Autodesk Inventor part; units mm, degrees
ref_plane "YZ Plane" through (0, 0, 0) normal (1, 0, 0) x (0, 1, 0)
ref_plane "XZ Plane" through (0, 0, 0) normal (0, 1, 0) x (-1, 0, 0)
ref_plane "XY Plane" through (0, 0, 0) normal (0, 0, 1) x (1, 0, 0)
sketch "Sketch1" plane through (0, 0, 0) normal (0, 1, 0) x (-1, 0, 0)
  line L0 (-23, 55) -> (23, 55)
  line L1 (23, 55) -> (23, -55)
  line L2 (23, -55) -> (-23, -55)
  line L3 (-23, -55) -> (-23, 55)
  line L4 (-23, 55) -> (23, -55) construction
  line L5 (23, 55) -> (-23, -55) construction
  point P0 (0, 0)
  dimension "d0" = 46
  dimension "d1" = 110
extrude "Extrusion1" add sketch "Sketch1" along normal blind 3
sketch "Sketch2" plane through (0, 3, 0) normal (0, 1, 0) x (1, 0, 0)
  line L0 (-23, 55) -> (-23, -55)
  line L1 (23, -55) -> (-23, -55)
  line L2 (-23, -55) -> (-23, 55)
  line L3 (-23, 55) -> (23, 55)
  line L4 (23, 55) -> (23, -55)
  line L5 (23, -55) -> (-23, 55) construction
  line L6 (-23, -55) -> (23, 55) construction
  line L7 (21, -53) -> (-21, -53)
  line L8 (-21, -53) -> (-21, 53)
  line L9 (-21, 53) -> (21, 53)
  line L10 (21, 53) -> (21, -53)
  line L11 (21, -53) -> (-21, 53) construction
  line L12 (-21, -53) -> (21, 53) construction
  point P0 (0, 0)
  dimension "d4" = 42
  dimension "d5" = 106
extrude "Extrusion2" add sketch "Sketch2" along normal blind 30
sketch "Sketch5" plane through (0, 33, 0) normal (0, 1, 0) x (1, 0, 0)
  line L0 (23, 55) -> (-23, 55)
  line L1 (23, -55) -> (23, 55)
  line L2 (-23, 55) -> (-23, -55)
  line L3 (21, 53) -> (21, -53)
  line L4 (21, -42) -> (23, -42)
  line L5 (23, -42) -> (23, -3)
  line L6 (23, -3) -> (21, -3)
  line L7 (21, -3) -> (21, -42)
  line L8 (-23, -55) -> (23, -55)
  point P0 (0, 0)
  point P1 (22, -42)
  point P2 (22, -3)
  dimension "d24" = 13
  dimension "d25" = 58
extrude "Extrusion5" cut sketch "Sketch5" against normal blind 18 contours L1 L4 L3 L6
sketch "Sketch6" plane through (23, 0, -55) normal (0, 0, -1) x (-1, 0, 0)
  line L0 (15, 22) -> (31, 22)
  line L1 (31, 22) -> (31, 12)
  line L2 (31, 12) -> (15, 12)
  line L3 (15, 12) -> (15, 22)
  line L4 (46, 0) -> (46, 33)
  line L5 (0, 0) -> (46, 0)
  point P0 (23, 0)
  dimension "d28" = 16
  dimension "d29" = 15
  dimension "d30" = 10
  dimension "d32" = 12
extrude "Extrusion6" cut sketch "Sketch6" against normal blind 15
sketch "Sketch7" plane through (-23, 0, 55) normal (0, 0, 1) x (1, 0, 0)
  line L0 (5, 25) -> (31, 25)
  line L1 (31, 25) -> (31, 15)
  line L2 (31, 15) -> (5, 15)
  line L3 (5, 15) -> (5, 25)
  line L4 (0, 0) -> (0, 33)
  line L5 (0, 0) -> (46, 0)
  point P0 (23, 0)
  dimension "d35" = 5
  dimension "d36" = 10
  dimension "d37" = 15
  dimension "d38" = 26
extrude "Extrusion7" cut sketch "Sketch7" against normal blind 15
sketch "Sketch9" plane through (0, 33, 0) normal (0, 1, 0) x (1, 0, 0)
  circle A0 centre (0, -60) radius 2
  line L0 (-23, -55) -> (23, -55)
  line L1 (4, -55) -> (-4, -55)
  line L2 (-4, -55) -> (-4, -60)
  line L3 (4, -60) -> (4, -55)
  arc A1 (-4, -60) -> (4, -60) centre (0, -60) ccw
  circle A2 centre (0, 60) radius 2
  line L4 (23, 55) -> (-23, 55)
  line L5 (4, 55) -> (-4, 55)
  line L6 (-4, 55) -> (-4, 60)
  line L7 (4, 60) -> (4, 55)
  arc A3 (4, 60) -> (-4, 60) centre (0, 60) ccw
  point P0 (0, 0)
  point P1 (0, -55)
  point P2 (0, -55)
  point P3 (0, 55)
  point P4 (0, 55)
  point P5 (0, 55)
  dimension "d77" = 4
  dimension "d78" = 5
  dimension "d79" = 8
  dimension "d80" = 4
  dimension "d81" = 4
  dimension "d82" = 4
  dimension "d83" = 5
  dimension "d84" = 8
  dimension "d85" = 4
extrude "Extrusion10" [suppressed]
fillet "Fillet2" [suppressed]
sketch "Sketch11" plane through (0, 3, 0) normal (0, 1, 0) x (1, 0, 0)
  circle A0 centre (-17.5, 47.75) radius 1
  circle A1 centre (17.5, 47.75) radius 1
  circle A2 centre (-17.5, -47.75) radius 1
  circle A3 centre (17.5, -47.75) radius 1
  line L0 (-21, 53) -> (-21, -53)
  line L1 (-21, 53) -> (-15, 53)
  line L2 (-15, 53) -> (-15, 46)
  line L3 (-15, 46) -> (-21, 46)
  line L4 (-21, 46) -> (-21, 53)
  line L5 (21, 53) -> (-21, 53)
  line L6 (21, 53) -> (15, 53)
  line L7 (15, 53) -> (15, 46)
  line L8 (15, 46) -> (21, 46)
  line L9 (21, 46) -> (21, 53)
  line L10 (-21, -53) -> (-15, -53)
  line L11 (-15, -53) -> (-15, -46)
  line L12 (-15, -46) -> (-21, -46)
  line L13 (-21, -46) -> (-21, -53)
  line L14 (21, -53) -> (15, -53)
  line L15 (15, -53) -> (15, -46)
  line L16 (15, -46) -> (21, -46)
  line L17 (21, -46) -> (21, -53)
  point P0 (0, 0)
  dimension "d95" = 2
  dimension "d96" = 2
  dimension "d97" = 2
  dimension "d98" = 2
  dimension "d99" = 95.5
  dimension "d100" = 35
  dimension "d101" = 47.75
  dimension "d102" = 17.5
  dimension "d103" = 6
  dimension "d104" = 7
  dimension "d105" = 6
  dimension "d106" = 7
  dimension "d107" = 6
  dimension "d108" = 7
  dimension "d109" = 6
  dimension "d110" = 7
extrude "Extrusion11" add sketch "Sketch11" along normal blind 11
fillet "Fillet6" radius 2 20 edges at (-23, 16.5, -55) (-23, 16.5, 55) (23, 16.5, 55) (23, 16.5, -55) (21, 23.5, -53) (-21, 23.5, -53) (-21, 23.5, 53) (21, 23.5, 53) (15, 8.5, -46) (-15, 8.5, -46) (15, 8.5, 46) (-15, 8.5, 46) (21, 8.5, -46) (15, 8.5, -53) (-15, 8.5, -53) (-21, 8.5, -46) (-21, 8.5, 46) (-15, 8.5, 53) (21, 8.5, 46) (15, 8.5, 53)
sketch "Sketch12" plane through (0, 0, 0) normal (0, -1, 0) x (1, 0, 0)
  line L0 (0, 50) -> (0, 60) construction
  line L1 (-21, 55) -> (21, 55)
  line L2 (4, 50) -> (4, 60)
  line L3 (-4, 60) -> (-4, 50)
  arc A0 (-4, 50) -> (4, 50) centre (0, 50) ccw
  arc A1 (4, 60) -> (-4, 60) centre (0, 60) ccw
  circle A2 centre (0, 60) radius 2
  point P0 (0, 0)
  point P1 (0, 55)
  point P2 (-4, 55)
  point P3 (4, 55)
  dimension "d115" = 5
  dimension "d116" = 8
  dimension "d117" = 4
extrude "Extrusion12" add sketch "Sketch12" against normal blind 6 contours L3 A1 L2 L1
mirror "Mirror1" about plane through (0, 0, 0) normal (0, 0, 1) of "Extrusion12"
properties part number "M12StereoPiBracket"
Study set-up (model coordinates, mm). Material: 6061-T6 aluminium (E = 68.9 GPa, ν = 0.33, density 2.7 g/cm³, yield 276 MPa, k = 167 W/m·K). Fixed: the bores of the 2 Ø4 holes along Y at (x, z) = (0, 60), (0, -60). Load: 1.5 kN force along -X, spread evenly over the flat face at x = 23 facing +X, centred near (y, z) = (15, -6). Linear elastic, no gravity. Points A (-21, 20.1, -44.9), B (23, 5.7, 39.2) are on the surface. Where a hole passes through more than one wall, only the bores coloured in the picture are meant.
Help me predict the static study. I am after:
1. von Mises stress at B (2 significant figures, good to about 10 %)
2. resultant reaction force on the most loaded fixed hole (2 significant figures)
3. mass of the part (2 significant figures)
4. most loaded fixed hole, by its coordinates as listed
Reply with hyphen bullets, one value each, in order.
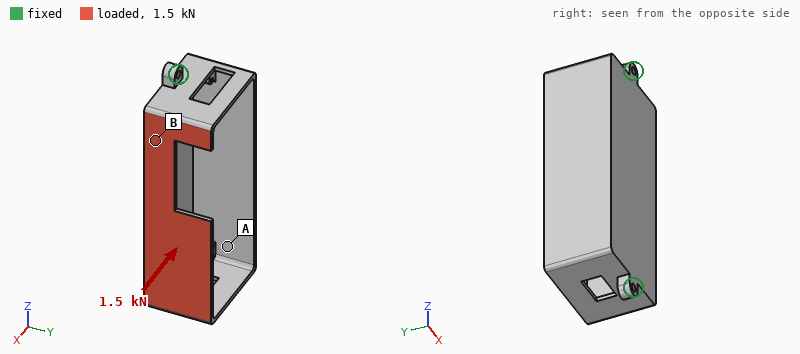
- 41 MPa
- 830 N
- 90 g
- (0, -60)
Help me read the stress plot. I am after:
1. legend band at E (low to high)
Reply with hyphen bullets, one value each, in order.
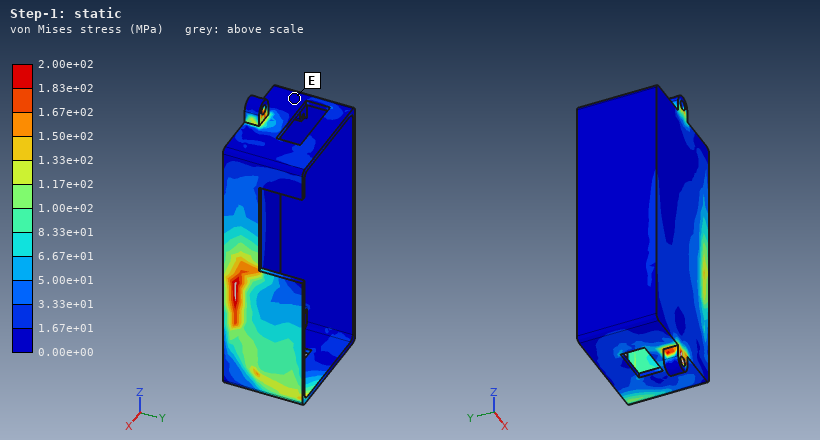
- 0.00e+00 to 1.67e+01 MPa
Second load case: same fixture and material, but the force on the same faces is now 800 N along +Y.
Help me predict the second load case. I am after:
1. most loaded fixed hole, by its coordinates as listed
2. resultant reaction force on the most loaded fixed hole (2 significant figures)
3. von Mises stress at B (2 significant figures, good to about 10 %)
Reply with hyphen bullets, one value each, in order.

- (0, -60)
- 440 N
- 30 MPa
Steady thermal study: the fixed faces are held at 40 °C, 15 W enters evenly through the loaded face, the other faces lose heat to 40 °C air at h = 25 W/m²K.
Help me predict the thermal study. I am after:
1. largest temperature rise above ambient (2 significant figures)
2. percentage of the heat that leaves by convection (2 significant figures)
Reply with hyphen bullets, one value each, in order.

- 17 K
- 31 %
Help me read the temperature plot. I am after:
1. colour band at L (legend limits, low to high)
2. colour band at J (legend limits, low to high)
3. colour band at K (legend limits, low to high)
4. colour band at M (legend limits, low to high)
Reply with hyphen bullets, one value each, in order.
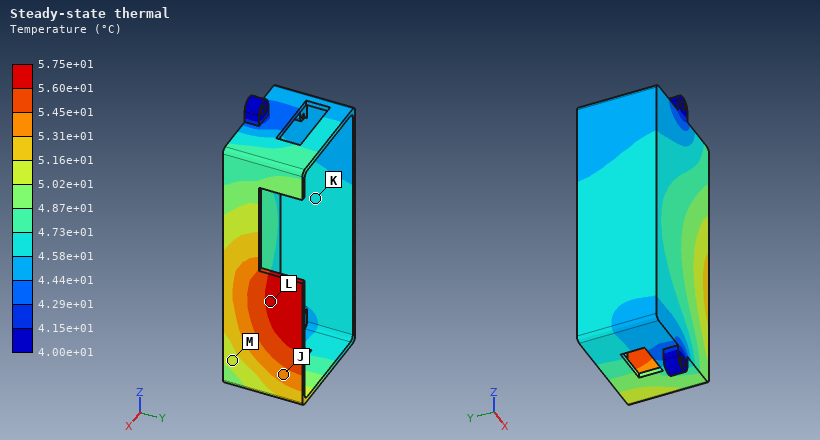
- 5.60e+01 to 5.75e+01 °C
- 5.31e+01 to 5.45e+01 °C
- 4.58e+01 to 4.73e+01 °C
- 5.02e+01 to 5.16e+01 °C
